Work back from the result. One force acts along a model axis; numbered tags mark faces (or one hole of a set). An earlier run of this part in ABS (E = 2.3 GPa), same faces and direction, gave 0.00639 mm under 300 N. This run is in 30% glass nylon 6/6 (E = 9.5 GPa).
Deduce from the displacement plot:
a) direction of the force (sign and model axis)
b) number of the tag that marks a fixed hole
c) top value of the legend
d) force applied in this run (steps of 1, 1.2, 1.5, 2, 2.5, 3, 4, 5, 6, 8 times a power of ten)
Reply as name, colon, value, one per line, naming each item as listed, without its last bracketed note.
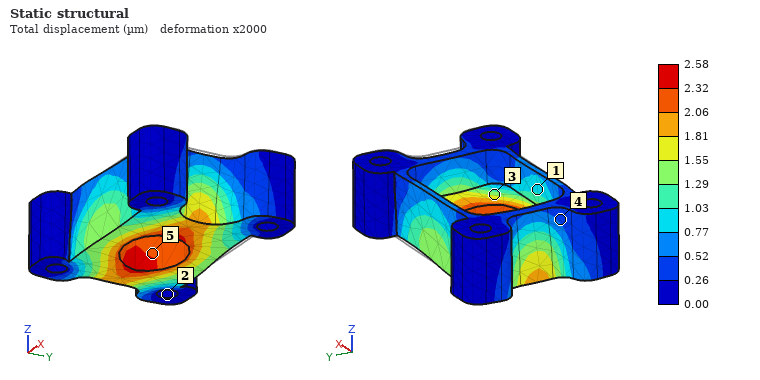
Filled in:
direction of the force: -X
number of the tag that marks a fixed hole: 2
top value of the legend: 2.58 µm
force applied in this run: 500 N
